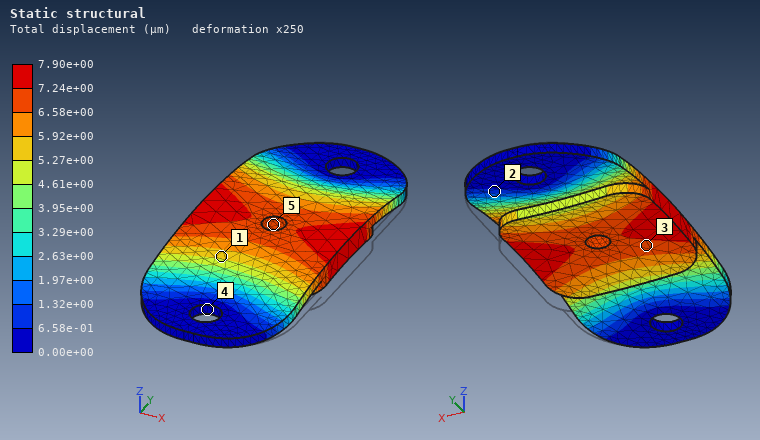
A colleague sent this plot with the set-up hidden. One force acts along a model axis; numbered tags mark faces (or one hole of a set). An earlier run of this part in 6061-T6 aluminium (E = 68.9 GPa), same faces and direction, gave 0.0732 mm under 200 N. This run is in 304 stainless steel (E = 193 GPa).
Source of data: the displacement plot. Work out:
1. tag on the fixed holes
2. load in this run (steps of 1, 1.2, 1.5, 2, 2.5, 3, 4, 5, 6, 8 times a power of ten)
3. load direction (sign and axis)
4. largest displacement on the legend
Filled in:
4
60 N
+Z
7.90e+00 µm
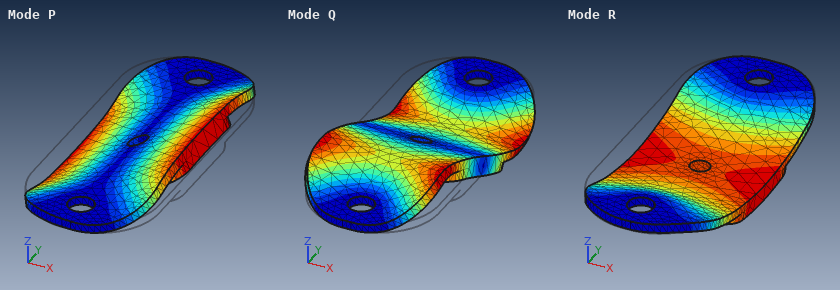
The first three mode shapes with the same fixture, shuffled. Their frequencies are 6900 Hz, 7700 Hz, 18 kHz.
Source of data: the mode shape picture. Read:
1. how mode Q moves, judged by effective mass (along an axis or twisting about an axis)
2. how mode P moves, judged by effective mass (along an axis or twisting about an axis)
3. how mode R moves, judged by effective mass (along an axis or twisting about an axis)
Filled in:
twisting about X
twisting about Y
along Z
